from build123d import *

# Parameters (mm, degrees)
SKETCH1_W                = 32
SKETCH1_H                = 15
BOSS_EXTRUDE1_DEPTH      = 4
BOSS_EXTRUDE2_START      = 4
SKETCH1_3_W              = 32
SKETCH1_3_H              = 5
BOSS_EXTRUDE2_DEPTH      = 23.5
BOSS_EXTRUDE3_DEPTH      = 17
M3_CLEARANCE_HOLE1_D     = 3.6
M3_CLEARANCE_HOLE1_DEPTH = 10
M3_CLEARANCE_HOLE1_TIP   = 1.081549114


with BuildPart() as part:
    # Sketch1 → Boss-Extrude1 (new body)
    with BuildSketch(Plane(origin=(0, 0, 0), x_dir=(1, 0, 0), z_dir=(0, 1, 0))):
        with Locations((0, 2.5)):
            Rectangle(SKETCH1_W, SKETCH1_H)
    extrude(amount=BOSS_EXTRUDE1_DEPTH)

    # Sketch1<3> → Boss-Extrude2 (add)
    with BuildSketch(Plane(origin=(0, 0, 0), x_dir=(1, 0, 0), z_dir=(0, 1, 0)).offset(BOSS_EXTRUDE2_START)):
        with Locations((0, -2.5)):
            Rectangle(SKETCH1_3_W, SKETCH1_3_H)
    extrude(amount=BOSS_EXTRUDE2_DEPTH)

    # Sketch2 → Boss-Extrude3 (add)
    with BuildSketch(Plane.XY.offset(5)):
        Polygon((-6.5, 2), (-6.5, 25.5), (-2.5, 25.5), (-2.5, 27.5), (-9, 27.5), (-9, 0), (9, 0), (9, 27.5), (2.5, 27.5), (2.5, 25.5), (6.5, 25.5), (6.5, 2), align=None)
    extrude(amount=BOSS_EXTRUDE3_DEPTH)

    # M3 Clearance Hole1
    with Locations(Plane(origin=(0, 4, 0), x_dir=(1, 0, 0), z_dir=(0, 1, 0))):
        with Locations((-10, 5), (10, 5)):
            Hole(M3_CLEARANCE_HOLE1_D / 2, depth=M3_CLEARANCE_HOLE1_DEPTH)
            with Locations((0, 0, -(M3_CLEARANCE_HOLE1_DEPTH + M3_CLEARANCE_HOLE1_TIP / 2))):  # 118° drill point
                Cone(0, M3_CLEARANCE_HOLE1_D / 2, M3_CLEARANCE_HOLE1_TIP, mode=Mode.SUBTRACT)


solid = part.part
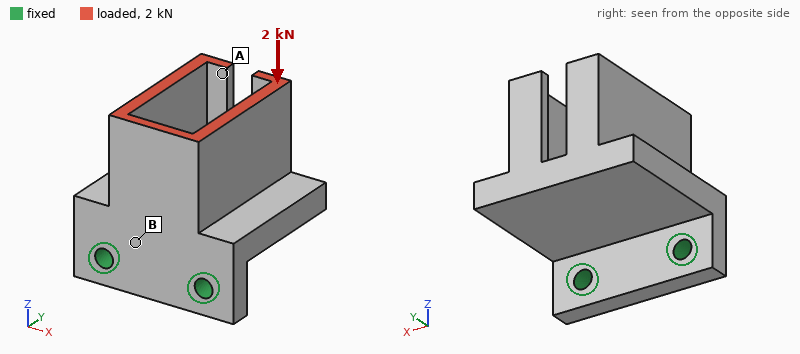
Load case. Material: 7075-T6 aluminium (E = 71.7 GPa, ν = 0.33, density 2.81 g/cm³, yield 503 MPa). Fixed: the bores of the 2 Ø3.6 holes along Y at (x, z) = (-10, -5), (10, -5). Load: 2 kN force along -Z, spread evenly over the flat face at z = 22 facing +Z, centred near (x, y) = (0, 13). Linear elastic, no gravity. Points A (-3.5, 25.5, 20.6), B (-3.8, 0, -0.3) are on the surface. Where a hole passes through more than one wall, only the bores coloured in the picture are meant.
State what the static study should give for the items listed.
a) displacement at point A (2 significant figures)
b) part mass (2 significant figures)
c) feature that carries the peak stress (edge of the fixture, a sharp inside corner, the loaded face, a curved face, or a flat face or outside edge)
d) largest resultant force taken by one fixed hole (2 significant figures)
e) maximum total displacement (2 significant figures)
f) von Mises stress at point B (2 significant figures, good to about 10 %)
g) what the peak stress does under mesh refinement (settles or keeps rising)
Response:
0.45 mm
24 g
edge of the fixture
1.0 kN
0.49 mm
180 MPa
keeps rising
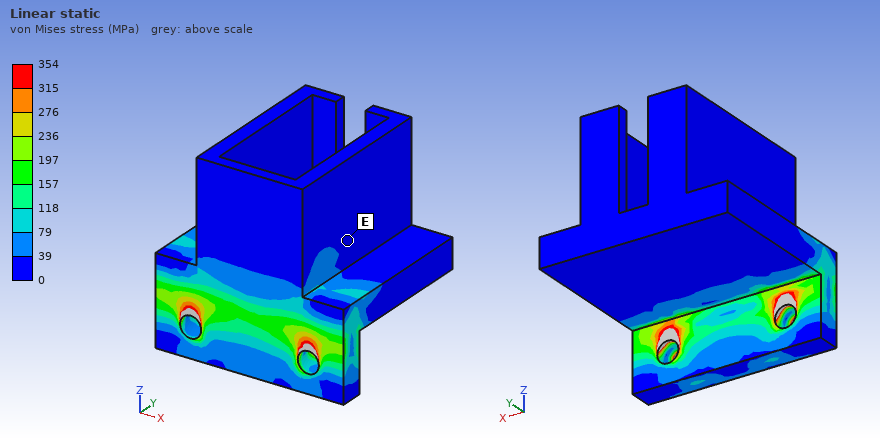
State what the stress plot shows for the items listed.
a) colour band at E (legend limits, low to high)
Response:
0 to 39 MPa
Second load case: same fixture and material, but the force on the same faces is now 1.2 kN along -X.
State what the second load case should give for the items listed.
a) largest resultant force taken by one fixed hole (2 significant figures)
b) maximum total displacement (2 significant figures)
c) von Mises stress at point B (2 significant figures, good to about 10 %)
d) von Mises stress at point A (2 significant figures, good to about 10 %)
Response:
1.7 kN
0.17 mm
17 MPa
19 MPa
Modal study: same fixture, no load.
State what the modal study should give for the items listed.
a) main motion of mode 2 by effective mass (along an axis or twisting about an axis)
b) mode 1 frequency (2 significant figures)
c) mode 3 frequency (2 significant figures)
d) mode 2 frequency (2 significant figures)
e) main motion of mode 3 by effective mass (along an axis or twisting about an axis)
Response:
along X
2500 Hz
7700 Hz
7300 Hz
along X
